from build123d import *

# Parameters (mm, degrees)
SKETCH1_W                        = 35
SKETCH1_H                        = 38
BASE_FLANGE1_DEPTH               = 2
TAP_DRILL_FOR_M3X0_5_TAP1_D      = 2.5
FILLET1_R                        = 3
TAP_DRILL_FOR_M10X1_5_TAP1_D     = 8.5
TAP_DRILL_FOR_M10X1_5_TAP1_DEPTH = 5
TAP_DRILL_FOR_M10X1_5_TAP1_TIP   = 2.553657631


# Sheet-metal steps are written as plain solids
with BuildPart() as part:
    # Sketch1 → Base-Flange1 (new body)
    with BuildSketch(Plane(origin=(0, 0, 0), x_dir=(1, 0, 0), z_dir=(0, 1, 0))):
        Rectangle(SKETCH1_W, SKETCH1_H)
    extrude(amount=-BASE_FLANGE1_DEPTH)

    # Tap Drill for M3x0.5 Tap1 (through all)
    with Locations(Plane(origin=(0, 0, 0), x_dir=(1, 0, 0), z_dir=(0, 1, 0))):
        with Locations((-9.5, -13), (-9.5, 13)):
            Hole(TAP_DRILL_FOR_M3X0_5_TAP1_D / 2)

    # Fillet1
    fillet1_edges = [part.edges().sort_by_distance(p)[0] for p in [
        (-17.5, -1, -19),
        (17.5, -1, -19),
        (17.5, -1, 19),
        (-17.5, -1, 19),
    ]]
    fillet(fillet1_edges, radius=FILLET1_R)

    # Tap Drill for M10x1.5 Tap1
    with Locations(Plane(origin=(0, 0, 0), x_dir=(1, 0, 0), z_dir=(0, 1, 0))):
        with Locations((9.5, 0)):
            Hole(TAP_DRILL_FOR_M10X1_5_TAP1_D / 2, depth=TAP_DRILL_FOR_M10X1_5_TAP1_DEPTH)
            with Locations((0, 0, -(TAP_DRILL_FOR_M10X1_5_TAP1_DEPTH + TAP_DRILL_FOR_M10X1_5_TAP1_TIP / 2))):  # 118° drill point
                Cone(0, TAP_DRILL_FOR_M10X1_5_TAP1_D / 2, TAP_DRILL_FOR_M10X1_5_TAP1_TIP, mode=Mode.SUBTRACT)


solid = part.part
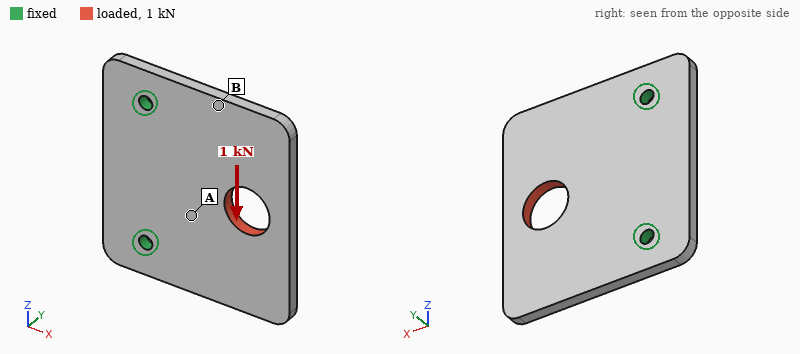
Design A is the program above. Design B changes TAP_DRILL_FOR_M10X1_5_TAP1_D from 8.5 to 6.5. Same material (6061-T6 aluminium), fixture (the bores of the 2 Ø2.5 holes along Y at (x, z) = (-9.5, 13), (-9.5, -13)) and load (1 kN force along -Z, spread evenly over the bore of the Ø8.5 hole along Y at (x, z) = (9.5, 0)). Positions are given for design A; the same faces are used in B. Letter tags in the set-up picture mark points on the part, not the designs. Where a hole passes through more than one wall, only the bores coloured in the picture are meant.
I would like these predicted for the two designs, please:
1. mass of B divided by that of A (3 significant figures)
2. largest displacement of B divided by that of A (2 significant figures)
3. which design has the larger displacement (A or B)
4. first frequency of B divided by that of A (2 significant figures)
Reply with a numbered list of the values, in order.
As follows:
1. 1.02
2. 0.92
3. A
4. 0.98
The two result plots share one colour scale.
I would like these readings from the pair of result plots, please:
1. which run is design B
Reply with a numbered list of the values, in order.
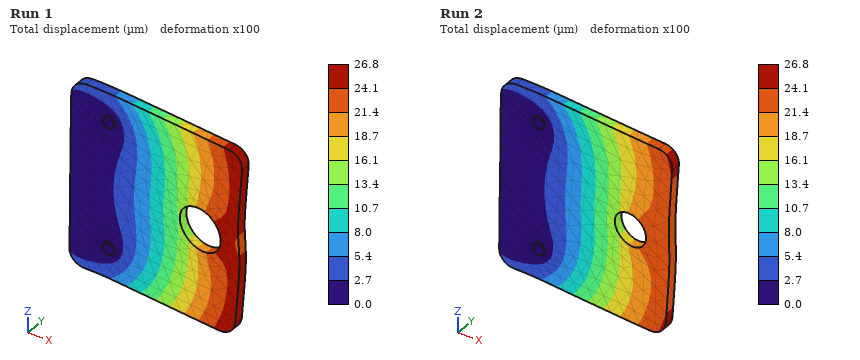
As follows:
1. Run 2
